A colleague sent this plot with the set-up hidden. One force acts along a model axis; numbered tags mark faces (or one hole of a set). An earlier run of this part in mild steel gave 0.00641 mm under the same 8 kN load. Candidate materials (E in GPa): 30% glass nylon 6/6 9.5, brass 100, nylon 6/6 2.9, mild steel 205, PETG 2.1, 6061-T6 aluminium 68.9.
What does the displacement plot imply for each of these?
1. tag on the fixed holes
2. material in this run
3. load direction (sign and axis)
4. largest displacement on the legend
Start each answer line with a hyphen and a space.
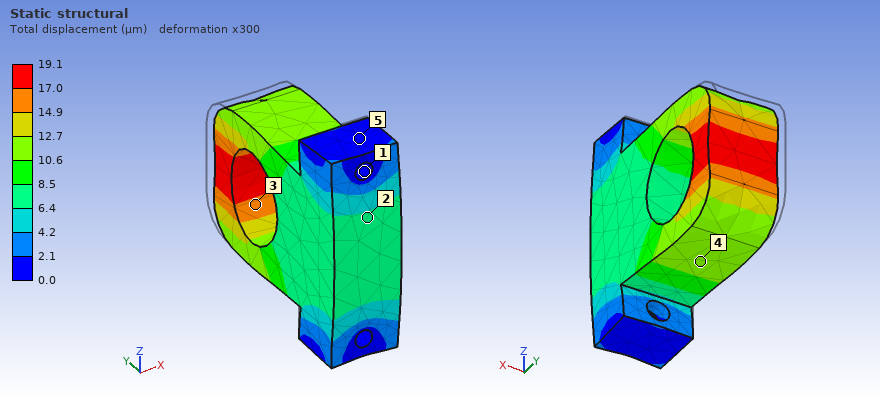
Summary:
- 1
- 6061-T6 aluminium
- -Y
- 19.1 µm
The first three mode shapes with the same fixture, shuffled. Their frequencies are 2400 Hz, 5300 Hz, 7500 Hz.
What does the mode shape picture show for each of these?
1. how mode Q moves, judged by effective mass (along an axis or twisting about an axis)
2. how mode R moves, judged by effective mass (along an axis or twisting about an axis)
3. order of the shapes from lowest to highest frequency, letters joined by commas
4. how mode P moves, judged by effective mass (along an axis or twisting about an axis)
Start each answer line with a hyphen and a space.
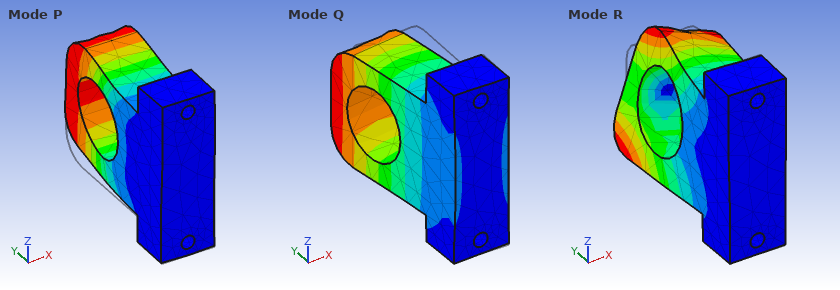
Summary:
- along X
- twisting about Y
- Q, P, R
- along Z
